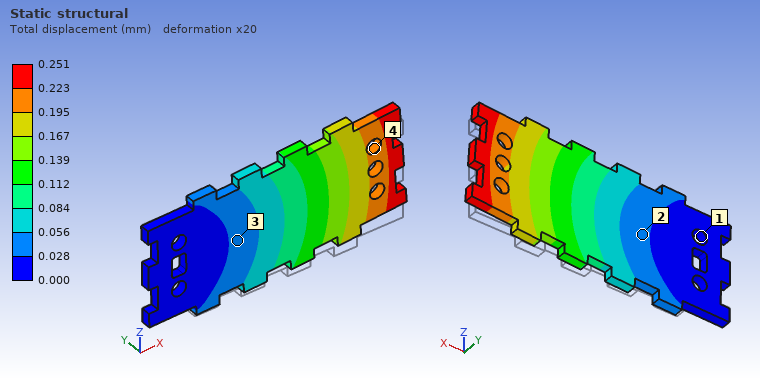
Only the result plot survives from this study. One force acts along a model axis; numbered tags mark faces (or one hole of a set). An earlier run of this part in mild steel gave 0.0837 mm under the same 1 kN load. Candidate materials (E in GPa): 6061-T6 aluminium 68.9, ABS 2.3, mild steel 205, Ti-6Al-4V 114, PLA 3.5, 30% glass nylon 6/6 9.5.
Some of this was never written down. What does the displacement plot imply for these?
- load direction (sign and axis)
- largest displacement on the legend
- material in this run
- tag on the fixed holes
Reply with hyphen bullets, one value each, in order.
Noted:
- +Z
- 0.251 mm
- 6061-T6 aluminium
- 1
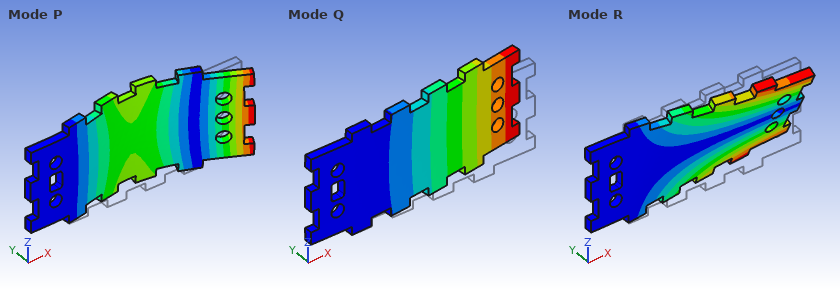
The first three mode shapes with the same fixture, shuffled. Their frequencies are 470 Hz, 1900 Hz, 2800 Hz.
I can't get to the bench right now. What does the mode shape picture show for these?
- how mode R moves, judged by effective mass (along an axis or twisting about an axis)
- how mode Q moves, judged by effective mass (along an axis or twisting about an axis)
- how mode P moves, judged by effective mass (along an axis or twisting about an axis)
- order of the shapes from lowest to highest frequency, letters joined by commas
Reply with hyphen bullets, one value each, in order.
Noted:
- twisting about X
- along Y
- along Y
- Q, R, P
